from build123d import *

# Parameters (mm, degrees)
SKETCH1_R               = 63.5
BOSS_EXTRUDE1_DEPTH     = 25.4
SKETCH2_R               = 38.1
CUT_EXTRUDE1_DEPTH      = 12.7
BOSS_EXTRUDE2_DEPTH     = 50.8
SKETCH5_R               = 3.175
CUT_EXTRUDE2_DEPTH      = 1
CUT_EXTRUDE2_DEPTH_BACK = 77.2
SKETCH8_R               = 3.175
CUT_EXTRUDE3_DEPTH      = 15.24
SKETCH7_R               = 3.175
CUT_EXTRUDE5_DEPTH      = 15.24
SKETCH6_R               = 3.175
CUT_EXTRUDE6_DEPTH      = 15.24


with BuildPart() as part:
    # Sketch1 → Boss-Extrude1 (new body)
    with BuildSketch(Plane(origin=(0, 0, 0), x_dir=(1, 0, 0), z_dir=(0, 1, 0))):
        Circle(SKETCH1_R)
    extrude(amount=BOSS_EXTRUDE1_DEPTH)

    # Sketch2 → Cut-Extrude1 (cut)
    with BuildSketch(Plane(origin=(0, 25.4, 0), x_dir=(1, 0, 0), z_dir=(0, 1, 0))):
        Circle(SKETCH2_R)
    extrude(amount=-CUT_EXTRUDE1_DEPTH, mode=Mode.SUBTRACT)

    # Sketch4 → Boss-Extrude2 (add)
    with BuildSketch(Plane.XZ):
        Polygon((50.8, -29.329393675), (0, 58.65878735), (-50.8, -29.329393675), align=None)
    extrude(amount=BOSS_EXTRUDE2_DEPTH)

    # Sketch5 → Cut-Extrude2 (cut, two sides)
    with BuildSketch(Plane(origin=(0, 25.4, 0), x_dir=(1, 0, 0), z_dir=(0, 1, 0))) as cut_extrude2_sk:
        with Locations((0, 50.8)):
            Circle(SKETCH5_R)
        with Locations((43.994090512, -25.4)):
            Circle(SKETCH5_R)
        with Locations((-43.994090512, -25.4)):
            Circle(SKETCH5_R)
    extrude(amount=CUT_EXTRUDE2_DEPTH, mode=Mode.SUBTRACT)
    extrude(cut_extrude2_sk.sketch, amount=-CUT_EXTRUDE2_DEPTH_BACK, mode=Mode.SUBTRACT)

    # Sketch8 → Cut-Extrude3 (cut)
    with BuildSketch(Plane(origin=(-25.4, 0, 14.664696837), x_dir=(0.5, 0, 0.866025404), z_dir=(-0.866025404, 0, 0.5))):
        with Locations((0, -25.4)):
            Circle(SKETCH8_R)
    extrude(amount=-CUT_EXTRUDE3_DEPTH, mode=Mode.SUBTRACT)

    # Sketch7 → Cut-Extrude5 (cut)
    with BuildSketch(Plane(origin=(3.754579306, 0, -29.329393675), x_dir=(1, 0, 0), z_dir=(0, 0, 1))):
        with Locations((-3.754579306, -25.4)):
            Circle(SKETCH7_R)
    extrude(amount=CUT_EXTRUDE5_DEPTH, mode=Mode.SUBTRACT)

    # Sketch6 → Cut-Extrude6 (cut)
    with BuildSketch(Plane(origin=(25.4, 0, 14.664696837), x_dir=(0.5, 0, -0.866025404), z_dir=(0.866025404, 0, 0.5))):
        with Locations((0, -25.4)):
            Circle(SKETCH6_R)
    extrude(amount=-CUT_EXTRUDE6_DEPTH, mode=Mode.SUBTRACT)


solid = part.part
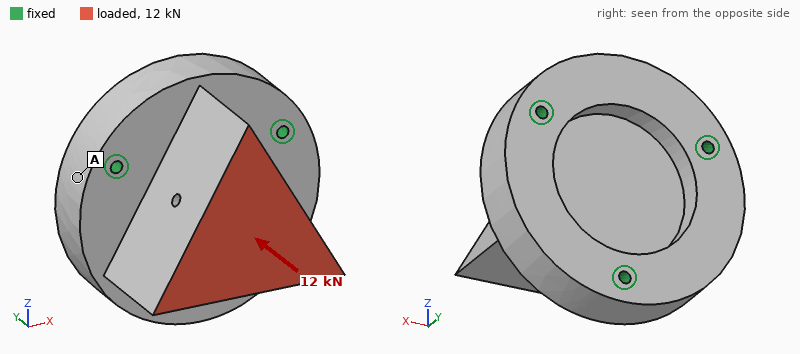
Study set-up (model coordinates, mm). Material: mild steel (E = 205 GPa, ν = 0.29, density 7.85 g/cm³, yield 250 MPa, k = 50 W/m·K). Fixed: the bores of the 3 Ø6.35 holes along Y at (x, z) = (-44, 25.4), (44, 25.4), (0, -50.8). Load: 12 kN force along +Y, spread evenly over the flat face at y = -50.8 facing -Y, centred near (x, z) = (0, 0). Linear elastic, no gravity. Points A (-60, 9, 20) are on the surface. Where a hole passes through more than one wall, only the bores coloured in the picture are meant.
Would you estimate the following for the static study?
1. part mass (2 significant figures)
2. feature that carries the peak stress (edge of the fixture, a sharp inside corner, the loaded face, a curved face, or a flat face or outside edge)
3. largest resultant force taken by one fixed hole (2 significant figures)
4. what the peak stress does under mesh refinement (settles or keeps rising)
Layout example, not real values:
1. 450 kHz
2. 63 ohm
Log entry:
1. 3.8 kg
2. edge of the fixture
3. 4.2 kN
4. keeps rising
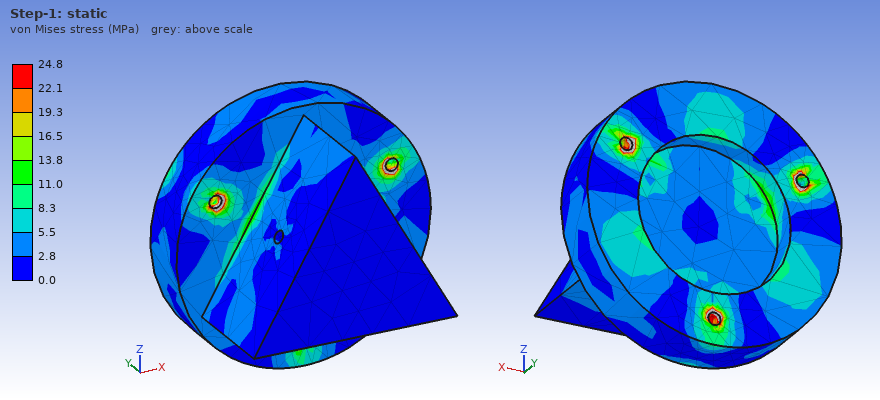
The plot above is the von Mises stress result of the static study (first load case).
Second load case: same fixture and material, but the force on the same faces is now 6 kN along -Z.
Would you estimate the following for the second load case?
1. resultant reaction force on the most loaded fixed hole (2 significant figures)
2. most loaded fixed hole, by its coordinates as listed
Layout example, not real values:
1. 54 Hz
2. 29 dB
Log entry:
1. 5.2 kN
2. (0, -50.8)
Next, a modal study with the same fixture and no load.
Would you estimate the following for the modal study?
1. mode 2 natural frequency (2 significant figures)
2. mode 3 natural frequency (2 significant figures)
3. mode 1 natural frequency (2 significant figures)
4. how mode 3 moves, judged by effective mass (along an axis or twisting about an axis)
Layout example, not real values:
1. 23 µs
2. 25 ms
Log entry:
1. 4600 Hz
2. 5900 Hz
3. 4600 Hz
4. along Y
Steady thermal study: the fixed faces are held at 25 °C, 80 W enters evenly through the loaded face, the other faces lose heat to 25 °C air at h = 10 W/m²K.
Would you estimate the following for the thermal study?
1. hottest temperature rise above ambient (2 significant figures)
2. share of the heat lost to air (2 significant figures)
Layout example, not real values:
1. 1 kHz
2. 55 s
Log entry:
1. 34 K
2. 8.5 %
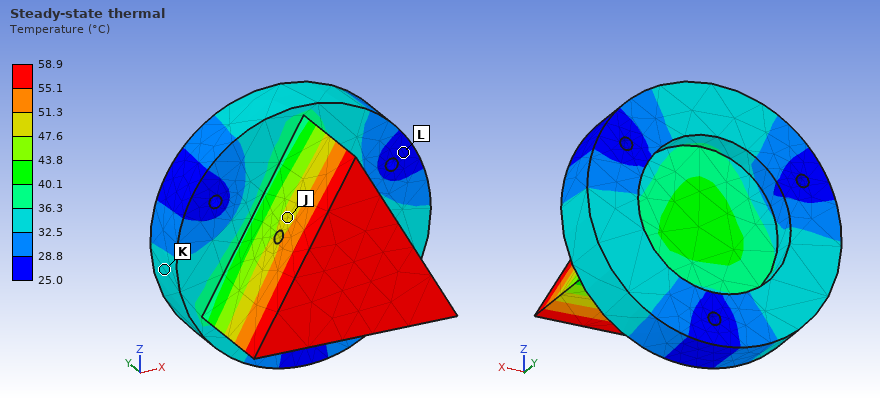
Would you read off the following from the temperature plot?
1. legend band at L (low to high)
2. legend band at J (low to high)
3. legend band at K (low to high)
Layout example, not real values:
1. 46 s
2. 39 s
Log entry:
1. 25.0 to 28.8 °C
2. 47.6 to 51.3 °C
3. 32.5 to 36.3 °C
